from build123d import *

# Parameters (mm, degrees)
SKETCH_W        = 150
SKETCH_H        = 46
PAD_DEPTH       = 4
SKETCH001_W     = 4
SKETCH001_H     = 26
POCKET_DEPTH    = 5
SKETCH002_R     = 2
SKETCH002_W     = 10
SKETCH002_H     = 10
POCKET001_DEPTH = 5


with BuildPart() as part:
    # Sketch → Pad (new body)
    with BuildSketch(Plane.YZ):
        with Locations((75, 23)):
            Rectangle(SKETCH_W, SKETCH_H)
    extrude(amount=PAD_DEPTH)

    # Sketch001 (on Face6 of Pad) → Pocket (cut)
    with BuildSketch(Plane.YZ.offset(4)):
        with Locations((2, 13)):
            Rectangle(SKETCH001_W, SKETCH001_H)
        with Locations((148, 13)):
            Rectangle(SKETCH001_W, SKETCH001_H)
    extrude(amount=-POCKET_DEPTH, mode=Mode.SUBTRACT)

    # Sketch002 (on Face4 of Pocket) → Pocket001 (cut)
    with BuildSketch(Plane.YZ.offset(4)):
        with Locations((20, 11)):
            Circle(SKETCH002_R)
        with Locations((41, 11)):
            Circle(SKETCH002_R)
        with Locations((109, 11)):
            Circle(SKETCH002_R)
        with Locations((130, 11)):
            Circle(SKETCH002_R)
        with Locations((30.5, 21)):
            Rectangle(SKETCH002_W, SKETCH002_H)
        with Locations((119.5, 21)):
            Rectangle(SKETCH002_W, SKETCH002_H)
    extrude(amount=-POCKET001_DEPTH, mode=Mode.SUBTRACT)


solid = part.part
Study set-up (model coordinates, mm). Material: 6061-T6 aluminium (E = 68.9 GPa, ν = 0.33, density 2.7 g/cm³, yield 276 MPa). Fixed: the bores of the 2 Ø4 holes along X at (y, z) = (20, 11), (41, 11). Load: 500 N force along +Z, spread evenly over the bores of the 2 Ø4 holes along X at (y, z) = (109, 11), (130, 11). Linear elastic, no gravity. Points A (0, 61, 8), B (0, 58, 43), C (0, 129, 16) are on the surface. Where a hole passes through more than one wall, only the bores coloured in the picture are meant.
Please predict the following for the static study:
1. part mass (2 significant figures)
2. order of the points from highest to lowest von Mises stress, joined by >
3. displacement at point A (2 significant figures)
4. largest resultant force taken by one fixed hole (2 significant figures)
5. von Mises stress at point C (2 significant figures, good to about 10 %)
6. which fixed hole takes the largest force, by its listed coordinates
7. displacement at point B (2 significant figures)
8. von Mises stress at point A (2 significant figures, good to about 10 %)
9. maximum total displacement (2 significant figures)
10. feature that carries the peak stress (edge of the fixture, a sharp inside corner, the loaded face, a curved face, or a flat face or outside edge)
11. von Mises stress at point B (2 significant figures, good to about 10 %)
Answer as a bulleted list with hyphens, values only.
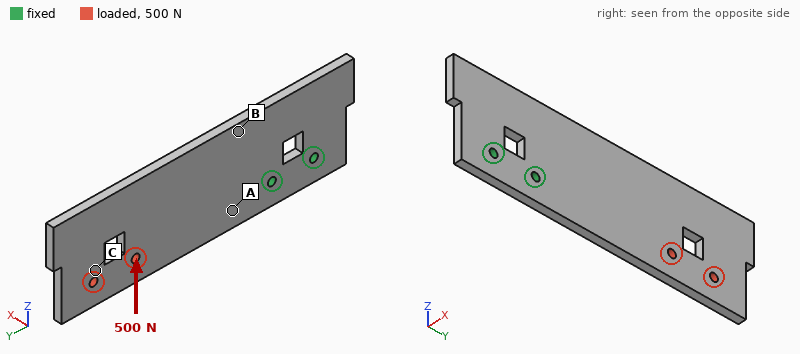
- 70 g
- B > A > C
- 0.030 mm
- 2.0 kN
- 6.5 MPa
- (41, 11)
- 0.048 mm
- 13 MPa
- 0.20 mm
- edge of the fixture
- 21 MPa
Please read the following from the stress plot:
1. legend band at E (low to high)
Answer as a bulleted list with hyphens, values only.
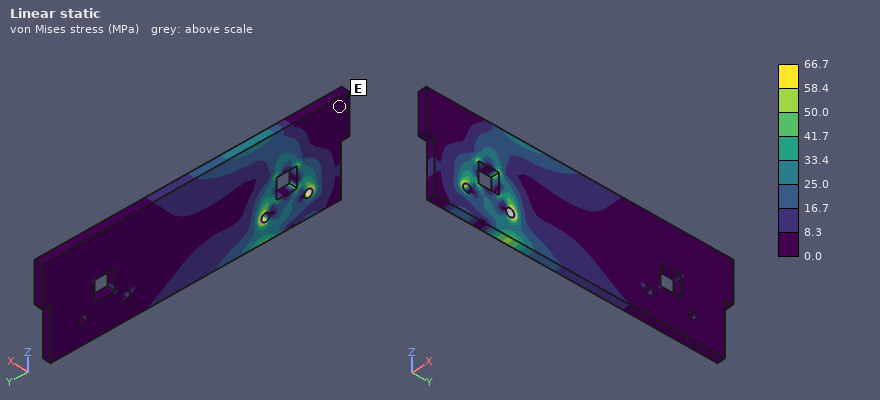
- 0.0 to 8.3 MPa
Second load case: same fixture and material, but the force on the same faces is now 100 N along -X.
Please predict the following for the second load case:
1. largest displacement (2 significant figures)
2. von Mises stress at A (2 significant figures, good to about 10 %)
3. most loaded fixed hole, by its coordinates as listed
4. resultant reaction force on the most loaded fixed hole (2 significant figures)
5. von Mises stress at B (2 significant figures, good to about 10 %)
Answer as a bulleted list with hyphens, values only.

- 1.7 mm
- 51 MPa
- (41, 11)
- 250 N
- 42 MPa
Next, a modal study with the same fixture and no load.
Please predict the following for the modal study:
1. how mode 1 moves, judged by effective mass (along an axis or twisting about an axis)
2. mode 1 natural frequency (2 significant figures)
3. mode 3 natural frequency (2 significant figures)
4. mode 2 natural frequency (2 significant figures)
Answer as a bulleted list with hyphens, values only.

- along X
- 270 Hz
- 1600 Hz
- 1100 Hz
